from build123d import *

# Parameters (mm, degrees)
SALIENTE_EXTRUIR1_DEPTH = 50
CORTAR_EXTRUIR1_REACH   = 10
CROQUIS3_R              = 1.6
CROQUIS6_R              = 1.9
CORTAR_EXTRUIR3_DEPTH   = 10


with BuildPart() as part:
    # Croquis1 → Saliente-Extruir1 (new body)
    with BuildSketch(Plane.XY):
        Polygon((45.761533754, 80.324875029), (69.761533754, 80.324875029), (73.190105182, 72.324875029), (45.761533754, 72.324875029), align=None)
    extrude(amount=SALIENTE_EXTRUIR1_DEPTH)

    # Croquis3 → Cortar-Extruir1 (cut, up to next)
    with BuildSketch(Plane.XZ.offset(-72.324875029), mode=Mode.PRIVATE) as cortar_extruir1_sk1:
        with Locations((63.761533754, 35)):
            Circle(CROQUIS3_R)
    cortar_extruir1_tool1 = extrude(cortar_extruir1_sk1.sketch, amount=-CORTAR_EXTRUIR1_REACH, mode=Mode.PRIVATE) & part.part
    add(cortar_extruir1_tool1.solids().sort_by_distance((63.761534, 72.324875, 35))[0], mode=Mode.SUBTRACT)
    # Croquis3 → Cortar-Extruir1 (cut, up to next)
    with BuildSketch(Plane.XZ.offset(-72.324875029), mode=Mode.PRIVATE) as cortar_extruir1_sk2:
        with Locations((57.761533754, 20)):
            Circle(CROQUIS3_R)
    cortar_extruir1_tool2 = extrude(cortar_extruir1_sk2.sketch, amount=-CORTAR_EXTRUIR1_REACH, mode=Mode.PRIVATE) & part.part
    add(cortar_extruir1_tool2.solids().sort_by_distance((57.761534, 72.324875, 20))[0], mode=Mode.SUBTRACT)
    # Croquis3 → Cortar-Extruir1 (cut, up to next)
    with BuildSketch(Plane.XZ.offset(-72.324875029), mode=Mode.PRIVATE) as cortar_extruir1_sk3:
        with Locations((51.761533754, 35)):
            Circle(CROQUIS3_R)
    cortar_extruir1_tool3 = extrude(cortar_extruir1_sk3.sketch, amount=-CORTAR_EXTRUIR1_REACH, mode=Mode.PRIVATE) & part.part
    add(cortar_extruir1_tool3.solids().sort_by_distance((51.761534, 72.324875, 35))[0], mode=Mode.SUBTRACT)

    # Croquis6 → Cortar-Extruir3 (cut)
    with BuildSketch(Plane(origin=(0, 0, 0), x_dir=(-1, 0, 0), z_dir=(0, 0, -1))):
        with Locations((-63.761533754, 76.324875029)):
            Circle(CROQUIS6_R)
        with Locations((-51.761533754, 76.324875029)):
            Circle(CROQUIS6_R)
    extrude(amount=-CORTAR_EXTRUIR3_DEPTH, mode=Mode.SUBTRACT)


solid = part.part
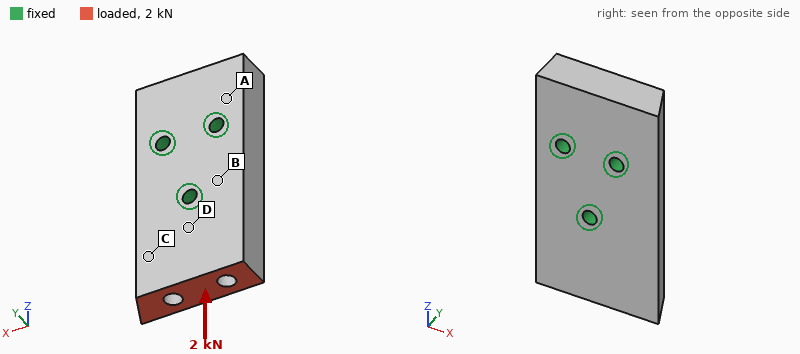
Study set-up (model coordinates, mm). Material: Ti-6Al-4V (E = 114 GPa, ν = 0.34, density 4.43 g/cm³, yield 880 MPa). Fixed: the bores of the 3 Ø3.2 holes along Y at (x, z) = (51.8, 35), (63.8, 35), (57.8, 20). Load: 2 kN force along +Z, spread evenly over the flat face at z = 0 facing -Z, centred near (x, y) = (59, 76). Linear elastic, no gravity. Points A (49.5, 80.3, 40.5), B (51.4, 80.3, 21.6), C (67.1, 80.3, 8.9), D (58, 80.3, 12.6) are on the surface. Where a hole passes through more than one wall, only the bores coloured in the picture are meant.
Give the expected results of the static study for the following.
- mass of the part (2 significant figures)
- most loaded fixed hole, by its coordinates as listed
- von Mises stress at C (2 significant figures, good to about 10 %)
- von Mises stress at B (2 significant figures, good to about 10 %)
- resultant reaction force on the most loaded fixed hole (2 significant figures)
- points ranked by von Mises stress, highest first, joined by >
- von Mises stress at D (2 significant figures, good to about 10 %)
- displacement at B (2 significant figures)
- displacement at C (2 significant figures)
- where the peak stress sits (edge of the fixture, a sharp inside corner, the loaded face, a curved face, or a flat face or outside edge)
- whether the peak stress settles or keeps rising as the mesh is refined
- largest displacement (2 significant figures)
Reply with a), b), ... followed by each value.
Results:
a) 44 g
b) (57.8, 20)
c) 10 MPa
d) 6.2 MPa
e) 1.3 kN
f) D > C > B > A
g) 15 MPa
h) 0.48 µm
i) 1.7 µm
j) edge of the fixture
k) keeps rising
l) 2.9 µm
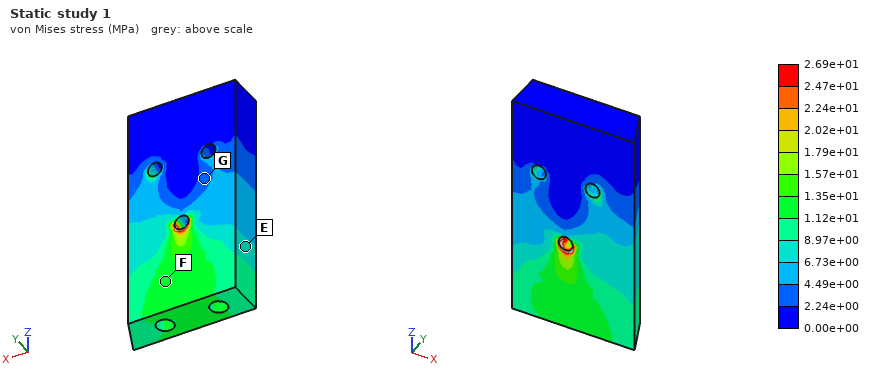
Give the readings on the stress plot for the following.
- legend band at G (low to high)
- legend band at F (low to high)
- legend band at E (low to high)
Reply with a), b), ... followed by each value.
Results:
a) 2.24e+00 to 4.49e+00 MPa
b) 1.12e+01 to 1.35e+01 MPa
c) 6.73e+00 to 8.97e+00 MPa
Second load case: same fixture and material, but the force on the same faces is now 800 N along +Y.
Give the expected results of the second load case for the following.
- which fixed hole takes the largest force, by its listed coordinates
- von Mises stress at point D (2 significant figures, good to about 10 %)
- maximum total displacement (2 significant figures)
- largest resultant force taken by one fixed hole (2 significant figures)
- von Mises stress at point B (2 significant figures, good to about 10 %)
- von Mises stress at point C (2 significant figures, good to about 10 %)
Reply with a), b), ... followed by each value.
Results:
a) (57.8, 20)
b) 40 MPa
c) 26 µm
d) 1.3 kN
e) 28 MPa
f) 27 MPa
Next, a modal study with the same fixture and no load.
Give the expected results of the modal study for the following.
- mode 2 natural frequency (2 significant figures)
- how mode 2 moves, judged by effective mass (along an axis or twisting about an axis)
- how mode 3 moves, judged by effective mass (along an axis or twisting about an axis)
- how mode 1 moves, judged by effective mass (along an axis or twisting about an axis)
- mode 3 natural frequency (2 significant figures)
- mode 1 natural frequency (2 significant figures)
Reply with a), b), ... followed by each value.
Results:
a) 18 kHz
b) twisting about Z
c) along X
d) along Y
e) 20 kHz
f) 13 kHz
